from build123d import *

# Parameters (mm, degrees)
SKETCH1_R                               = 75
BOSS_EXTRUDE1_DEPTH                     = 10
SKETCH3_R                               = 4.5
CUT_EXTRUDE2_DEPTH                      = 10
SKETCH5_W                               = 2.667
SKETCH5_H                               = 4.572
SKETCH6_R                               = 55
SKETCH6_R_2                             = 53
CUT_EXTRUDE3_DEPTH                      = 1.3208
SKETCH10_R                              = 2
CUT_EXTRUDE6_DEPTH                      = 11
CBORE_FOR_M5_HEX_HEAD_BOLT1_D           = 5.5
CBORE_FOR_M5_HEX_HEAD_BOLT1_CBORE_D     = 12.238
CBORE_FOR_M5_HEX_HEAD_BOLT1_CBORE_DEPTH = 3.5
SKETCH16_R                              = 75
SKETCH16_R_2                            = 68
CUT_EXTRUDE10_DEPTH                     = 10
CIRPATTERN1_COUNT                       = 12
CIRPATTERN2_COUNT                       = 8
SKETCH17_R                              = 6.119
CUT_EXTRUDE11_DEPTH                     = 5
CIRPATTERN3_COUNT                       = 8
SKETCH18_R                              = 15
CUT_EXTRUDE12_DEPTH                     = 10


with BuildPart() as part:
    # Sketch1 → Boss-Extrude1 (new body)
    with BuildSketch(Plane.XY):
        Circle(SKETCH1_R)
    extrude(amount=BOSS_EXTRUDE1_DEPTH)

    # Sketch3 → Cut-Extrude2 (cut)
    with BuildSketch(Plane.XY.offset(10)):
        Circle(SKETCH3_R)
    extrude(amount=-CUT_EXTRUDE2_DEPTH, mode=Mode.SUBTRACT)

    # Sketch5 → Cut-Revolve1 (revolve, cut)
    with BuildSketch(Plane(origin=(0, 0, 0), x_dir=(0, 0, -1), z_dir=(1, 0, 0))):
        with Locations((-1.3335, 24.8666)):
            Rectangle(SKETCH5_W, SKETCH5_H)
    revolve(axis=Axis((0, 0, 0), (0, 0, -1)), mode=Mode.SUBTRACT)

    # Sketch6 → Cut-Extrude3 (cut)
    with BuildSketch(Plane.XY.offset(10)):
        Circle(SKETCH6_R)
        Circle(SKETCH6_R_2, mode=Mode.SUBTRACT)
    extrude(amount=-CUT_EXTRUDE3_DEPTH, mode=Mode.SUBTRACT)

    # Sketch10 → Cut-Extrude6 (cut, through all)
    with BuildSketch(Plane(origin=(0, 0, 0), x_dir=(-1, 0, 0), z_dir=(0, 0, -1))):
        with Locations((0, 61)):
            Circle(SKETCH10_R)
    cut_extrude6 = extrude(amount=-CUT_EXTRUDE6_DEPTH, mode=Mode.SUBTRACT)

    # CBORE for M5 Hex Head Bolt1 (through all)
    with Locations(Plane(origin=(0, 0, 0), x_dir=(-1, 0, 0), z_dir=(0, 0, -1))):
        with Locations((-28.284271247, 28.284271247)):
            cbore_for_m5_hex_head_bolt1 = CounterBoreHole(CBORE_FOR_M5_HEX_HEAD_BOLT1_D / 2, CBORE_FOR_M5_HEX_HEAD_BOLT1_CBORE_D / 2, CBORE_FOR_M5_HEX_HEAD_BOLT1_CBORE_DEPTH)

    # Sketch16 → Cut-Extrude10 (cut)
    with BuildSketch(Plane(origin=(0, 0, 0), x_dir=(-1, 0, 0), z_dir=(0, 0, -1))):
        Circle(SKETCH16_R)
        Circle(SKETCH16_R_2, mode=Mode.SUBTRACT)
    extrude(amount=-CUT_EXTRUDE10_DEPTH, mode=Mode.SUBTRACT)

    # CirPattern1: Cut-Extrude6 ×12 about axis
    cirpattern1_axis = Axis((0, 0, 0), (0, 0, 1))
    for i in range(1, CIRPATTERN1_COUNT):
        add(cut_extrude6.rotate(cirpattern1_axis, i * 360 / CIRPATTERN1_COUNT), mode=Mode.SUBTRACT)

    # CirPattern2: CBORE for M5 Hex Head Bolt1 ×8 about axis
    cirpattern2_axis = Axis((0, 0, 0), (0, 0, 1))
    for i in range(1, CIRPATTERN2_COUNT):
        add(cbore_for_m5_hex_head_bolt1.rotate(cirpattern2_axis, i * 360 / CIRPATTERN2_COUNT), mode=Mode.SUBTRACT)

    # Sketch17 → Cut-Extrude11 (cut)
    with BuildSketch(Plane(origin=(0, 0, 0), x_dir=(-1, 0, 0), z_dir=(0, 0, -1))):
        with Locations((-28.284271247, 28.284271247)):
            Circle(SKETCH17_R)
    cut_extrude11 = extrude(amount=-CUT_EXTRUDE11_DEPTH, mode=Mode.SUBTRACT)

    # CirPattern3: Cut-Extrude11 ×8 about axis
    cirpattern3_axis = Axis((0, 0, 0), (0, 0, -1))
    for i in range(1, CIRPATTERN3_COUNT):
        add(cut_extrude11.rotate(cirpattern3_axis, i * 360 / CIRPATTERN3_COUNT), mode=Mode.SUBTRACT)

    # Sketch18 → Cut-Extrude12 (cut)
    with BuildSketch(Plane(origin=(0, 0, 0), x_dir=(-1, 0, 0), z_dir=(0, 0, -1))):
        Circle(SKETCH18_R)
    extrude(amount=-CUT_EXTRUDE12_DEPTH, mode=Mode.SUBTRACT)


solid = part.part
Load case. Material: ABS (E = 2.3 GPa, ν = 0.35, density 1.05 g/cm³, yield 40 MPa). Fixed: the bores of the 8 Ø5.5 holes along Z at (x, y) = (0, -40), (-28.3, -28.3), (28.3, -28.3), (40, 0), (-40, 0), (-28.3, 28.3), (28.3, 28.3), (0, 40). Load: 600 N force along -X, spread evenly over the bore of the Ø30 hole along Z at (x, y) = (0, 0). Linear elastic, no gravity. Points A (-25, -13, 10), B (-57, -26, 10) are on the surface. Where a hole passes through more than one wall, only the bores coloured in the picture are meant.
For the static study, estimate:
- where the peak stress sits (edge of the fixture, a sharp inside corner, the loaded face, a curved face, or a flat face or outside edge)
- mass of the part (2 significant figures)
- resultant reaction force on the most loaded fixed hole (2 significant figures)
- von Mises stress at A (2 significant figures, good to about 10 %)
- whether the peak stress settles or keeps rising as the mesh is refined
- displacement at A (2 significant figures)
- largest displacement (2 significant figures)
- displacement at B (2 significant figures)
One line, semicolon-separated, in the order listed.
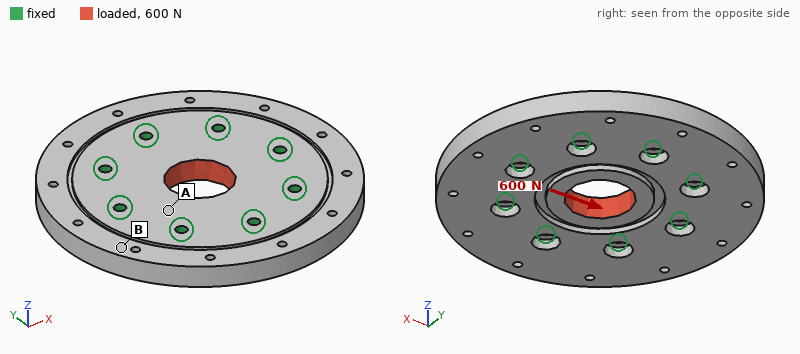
edge of the fixture; 130 g; 110 N; 0.42 MPa; keeps rising; 5.0 µm; 13 µm; 5.4 µm
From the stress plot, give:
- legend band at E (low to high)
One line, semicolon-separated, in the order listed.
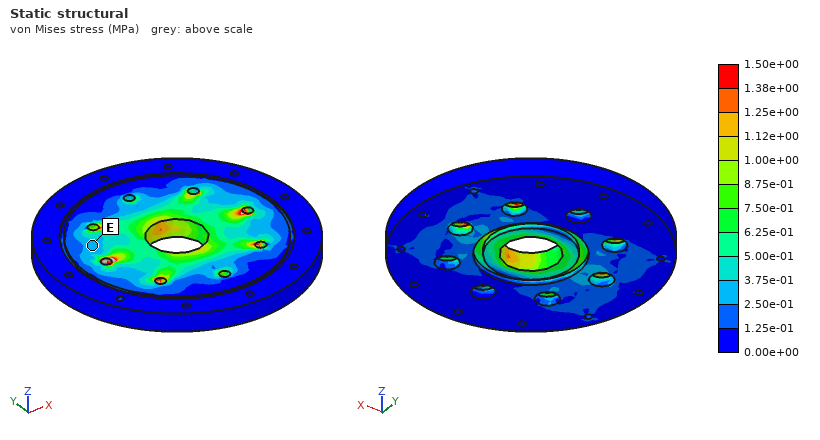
2.50e-01 to 3.75e-01 MPa
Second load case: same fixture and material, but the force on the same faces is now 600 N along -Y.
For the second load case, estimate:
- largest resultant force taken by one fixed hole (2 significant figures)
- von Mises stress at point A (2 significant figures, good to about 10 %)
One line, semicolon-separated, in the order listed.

110 N; 0.53 MPa
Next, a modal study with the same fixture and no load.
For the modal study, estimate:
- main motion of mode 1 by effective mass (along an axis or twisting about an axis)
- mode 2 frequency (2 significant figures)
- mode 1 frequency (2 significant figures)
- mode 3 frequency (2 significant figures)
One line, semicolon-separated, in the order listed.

along Z; 1800 Hz; 1600 Hz; 1800 Hz
